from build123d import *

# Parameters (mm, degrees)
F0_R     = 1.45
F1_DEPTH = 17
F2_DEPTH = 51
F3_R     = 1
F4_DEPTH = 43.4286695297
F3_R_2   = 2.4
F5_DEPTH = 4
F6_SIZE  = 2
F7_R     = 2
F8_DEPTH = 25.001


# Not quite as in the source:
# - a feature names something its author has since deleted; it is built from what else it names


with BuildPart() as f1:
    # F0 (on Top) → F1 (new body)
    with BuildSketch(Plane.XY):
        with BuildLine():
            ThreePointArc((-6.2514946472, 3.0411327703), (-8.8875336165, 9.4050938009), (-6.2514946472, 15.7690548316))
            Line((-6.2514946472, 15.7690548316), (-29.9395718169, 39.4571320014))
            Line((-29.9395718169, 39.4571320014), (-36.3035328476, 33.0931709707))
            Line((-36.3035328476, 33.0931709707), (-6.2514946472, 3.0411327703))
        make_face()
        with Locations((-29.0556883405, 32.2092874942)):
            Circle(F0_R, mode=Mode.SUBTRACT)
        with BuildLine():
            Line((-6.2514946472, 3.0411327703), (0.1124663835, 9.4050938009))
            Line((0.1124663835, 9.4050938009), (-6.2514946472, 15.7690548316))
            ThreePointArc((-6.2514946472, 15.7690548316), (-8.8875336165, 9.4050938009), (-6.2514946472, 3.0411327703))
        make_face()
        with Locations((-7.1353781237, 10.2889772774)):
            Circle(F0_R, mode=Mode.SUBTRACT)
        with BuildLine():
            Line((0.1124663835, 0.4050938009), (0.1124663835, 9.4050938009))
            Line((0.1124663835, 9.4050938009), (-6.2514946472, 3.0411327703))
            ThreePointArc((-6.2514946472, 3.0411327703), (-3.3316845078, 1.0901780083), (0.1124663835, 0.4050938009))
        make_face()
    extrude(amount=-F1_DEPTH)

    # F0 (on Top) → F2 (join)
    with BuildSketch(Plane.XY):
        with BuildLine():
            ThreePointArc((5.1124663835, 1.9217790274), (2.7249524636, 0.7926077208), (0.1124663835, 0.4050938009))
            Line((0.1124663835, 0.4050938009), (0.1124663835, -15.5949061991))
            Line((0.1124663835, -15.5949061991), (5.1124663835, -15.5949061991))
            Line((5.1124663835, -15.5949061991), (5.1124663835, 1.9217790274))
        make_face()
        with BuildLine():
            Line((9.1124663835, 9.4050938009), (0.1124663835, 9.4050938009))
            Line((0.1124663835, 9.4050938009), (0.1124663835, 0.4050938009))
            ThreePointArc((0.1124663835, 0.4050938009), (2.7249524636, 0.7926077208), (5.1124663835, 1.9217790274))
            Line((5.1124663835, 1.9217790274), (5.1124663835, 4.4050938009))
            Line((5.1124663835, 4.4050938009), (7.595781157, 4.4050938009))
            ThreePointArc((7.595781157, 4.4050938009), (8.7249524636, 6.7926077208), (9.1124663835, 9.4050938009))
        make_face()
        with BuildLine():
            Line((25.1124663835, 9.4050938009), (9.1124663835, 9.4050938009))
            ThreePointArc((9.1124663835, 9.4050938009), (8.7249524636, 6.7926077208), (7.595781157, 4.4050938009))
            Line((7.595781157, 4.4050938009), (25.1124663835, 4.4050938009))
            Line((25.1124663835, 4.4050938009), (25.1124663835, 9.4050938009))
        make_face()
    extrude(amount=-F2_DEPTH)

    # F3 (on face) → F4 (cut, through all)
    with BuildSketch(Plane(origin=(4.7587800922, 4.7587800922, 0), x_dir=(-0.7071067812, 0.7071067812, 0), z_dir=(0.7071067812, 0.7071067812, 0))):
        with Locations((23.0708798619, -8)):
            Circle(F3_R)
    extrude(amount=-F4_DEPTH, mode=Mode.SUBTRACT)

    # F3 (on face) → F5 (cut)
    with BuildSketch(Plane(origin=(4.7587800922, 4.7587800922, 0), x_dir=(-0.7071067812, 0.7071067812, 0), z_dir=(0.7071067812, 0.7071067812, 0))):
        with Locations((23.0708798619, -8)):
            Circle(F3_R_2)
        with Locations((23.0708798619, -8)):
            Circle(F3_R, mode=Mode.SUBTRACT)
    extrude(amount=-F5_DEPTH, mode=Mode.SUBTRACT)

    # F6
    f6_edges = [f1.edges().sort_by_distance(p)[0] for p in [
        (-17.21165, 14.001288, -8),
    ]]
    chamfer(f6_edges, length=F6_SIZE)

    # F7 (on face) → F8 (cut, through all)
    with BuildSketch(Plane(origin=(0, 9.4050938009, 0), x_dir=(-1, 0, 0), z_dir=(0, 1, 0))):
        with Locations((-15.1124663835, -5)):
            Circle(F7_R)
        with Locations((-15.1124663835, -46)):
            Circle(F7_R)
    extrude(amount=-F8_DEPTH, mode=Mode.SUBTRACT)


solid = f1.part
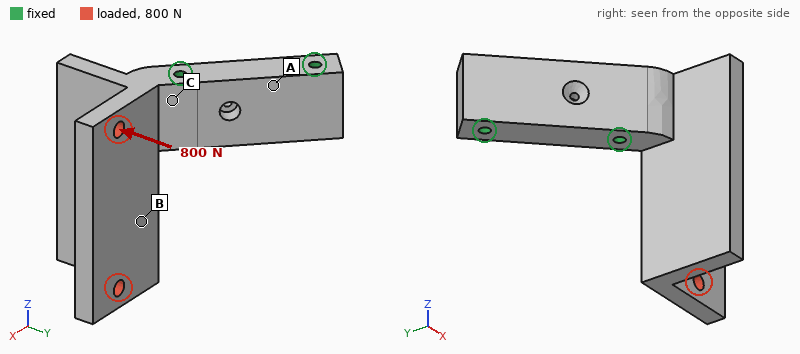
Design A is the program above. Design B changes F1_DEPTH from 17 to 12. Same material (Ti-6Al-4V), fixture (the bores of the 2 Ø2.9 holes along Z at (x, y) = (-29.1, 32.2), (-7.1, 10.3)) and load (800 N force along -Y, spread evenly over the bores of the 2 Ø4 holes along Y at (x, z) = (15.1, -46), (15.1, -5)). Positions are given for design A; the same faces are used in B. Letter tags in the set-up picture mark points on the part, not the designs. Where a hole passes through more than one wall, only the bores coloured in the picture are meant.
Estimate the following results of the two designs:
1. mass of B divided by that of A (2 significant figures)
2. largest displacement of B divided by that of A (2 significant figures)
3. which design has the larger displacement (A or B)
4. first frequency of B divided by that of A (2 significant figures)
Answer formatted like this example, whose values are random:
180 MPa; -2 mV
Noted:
0.89; 1.5; B; 0.75
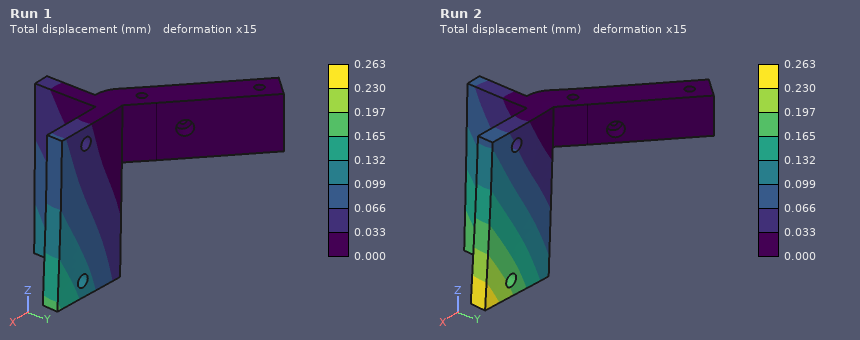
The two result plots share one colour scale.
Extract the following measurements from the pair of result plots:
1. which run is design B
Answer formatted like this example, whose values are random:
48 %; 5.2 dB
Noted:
Run 2
